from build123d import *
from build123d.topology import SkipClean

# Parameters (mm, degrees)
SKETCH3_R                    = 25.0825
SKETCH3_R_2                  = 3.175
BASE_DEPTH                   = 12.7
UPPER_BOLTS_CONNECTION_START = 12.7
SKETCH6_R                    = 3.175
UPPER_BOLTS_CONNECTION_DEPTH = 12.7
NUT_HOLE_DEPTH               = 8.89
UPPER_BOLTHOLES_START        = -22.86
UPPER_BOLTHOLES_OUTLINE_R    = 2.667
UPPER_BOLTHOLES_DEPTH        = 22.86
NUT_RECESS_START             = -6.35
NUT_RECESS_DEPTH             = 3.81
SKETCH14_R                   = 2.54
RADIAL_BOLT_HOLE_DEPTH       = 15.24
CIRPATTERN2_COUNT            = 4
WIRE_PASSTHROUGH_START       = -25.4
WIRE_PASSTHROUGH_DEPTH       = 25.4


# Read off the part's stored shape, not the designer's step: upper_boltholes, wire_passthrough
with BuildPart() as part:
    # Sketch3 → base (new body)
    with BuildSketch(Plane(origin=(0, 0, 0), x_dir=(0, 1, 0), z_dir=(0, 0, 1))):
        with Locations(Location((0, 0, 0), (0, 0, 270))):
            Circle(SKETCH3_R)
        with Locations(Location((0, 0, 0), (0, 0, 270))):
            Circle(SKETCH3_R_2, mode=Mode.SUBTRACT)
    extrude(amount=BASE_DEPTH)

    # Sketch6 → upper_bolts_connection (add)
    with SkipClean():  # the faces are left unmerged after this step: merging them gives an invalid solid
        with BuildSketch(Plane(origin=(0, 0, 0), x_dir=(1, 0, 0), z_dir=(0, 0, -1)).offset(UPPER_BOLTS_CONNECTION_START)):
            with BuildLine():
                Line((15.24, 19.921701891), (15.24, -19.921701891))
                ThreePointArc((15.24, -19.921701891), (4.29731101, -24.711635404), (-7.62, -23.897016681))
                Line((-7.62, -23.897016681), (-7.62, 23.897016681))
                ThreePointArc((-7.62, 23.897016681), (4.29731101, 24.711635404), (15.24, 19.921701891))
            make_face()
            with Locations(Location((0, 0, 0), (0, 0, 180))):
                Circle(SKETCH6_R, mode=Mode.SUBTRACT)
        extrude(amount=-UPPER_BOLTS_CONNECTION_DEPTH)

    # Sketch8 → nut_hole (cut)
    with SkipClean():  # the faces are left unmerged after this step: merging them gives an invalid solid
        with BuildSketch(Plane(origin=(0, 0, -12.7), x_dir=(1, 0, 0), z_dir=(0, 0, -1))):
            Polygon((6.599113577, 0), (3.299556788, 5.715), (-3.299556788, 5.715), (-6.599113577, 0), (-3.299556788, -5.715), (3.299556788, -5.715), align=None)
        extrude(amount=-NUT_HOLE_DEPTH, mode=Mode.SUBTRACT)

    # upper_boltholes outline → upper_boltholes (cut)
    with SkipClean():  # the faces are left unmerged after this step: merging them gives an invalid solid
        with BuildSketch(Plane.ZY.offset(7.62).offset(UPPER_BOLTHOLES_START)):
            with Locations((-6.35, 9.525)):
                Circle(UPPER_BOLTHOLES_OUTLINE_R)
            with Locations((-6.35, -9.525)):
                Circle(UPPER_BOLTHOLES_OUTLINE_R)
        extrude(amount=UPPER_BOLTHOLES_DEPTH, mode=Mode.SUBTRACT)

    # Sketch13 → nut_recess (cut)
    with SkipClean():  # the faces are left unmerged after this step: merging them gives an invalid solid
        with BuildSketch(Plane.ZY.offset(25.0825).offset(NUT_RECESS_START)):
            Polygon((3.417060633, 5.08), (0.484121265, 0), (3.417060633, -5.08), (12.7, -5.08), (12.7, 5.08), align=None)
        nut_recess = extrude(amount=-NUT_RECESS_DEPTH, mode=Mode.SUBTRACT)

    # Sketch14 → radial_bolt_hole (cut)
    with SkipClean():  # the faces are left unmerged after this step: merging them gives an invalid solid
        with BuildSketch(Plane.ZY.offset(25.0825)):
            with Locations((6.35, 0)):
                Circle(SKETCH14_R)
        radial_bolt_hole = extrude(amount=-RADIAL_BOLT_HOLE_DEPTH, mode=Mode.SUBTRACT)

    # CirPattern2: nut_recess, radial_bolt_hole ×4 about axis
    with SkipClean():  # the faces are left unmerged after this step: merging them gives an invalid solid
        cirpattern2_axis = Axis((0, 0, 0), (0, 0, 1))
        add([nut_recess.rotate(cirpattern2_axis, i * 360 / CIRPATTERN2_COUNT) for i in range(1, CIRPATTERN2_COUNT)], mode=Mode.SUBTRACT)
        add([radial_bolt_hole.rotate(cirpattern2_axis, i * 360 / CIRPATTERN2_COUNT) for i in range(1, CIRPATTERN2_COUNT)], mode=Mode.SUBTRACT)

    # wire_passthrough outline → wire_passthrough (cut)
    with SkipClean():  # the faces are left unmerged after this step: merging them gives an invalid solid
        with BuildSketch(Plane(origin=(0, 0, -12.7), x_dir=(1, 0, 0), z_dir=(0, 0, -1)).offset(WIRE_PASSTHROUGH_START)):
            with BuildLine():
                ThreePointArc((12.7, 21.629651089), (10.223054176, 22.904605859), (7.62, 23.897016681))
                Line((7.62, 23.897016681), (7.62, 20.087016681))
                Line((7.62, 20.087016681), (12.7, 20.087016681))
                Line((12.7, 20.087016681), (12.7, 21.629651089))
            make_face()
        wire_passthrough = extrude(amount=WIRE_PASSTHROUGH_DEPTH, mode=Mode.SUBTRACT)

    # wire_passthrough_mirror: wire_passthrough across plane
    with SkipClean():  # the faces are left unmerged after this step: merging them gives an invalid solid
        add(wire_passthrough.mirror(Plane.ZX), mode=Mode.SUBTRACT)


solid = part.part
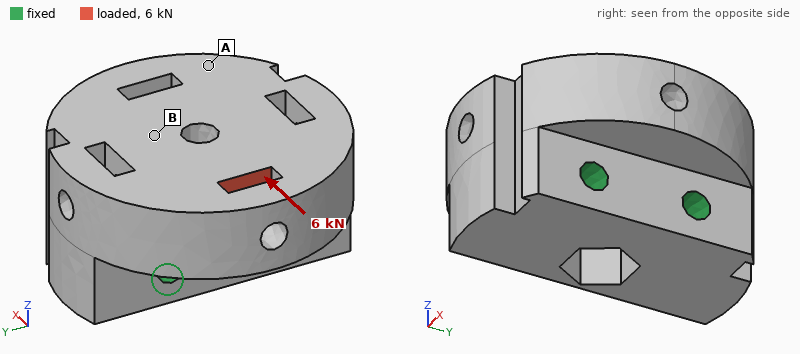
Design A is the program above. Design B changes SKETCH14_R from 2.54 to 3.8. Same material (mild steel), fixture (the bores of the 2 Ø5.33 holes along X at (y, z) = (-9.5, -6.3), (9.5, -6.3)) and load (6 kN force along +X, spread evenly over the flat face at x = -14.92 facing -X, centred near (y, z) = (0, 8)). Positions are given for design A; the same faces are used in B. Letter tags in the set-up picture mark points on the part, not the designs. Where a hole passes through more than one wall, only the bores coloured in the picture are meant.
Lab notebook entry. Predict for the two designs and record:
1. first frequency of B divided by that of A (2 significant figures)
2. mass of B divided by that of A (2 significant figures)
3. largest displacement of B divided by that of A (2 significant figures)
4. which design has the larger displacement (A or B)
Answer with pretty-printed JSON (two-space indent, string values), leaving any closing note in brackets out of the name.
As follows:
{
  "first frequency of B divided by that of A": "1.00",
  "mass of B divided by that of A": "0.97",
  "largest displacement of B divided by that of A": "1.2",
  "which design has the larger displacement": "B"
}
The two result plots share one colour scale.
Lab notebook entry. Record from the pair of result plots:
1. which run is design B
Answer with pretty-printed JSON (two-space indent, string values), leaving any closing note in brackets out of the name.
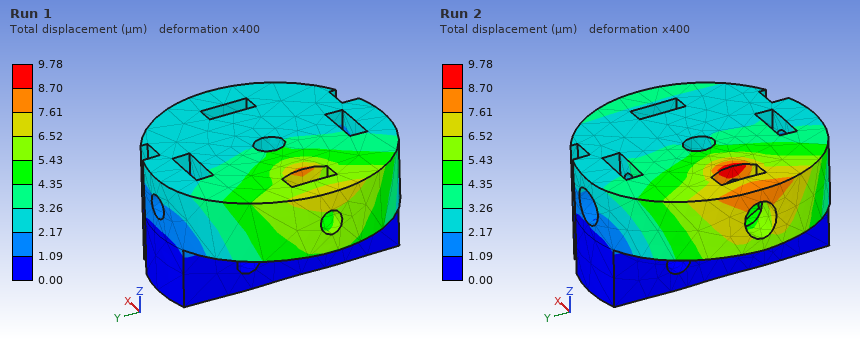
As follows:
{
  "which run is design B": "Run 2"
}
